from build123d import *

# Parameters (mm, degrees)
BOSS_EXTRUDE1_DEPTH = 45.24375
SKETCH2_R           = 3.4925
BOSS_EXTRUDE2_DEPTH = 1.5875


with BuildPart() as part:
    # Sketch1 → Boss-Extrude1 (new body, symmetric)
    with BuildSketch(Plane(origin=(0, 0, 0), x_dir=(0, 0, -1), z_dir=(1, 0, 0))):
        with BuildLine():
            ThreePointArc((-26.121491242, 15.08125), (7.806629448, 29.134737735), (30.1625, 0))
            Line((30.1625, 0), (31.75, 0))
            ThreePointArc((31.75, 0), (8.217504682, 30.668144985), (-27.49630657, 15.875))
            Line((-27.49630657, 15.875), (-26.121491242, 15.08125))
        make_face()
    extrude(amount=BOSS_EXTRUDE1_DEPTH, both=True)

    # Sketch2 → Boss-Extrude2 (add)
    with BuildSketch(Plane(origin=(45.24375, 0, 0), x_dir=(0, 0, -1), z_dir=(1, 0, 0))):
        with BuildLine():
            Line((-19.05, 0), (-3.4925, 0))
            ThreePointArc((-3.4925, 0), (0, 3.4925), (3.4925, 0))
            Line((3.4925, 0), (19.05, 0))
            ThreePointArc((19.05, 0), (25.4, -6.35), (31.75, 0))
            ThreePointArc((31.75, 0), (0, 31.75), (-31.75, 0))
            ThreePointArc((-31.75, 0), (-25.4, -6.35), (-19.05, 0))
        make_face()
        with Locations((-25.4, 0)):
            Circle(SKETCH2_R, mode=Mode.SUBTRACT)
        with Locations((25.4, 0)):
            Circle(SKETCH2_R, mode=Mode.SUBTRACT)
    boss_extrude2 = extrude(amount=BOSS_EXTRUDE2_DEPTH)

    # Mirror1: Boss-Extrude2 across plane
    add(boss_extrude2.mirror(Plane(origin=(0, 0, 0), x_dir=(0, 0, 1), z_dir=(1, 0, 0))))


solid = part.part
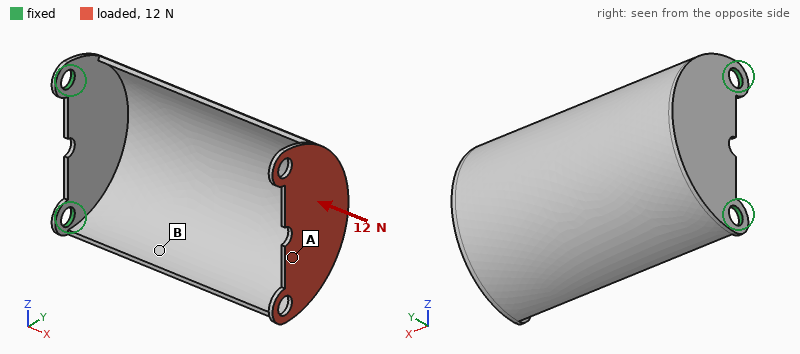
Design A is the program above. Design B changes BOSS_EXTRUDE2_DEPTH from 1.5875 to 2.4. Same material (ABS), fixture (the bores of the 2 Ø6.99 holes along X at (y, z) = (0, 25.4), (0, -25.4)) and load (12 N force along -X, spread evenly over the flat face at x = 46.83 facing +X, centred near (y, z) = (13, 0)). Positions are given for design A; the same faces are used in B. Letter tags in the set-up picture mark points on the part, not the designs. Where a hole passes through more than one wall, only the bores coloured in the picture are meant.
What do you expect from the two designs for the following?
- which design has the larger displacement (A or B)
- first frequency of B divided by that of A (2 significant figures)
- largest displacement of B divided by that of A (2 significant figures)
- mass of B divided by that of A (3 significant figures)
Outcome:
A
1.3
0.46
1.16
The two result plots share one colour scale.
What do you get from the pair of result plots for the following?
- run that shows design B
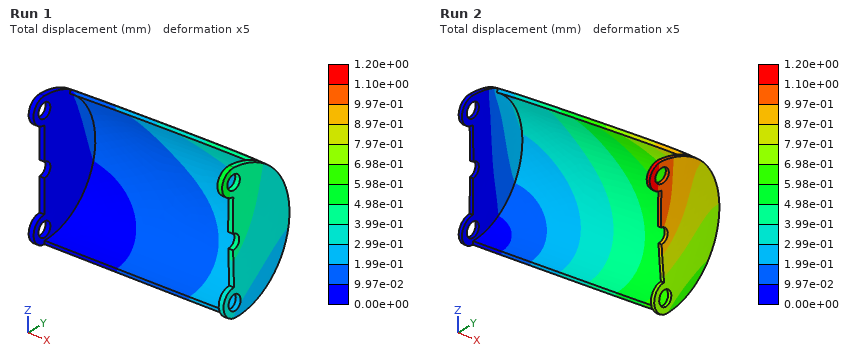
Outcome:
Run 1
